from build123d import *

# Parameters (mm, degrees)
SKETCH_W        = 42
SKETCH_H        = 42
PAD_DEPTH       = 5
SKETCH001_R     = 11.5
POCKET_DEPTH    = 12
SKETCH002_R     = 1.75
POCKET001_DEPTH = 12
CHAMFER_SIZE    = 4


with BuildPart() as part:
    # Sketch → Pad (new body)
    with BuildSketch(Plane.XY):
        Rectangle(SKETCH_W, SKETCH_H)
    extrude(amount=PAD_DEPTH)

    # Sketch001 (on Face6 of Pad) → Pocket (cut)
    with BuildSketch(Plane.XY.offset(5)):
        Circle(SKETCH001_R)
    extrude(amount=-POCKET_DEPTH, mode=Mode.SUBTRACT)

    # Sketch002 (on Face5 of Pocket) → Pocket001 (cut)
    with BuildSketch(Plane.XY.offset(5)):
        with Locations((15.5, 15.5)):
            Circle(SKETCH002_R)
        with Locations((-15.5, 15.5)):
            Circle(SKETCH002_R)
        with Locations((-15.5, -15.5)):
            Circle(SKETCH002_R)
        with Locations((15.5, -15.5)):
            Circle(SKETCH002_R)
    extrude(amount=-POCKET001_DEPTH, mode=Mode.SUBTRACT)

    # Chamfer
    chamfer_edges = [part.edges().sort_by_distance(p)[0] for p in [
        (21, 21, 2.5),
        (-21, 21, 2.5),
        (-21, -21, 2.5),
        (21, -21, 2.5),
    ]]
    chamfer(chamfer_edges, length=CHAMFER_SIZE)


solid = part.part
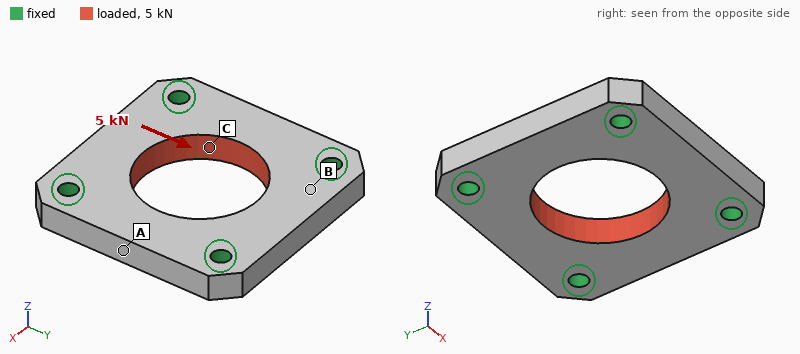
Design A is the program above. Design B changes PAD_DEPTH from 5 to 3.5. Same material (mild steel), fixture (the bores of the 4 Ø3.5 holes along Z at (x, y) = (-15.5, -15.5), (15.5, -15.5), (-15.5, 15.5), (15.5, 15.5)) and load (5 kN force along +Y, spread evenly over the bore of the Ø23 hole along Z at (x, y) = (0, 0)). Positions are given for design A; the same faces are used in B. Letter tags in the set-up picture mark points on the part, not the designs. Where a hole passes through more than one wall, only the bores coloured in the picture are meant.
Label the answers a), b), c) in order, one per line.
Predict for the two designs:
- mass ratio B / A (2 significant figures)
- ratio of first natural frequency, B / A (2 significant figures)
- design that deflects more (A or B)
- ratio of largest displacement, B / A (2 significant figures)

a) 0.70
b) 0.78
c) B
d) 1.4
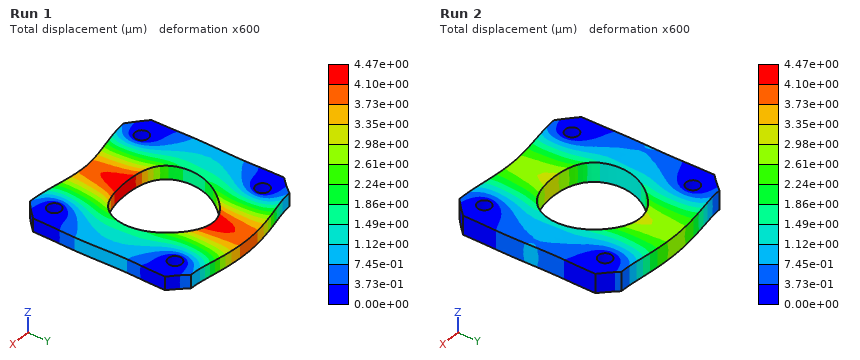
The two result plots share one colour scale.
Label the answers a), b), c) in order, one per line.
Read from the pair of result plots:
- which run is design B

a) Run 1
